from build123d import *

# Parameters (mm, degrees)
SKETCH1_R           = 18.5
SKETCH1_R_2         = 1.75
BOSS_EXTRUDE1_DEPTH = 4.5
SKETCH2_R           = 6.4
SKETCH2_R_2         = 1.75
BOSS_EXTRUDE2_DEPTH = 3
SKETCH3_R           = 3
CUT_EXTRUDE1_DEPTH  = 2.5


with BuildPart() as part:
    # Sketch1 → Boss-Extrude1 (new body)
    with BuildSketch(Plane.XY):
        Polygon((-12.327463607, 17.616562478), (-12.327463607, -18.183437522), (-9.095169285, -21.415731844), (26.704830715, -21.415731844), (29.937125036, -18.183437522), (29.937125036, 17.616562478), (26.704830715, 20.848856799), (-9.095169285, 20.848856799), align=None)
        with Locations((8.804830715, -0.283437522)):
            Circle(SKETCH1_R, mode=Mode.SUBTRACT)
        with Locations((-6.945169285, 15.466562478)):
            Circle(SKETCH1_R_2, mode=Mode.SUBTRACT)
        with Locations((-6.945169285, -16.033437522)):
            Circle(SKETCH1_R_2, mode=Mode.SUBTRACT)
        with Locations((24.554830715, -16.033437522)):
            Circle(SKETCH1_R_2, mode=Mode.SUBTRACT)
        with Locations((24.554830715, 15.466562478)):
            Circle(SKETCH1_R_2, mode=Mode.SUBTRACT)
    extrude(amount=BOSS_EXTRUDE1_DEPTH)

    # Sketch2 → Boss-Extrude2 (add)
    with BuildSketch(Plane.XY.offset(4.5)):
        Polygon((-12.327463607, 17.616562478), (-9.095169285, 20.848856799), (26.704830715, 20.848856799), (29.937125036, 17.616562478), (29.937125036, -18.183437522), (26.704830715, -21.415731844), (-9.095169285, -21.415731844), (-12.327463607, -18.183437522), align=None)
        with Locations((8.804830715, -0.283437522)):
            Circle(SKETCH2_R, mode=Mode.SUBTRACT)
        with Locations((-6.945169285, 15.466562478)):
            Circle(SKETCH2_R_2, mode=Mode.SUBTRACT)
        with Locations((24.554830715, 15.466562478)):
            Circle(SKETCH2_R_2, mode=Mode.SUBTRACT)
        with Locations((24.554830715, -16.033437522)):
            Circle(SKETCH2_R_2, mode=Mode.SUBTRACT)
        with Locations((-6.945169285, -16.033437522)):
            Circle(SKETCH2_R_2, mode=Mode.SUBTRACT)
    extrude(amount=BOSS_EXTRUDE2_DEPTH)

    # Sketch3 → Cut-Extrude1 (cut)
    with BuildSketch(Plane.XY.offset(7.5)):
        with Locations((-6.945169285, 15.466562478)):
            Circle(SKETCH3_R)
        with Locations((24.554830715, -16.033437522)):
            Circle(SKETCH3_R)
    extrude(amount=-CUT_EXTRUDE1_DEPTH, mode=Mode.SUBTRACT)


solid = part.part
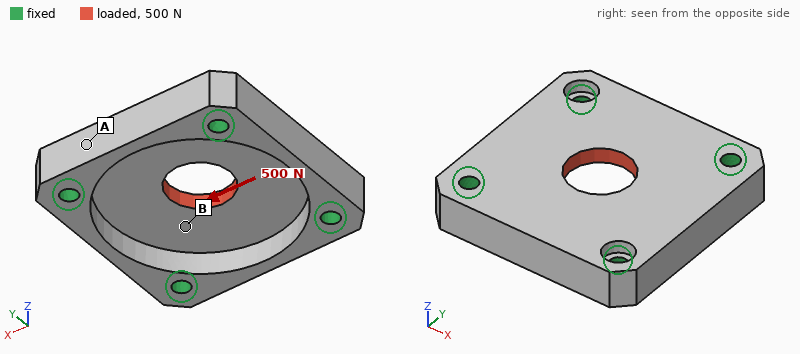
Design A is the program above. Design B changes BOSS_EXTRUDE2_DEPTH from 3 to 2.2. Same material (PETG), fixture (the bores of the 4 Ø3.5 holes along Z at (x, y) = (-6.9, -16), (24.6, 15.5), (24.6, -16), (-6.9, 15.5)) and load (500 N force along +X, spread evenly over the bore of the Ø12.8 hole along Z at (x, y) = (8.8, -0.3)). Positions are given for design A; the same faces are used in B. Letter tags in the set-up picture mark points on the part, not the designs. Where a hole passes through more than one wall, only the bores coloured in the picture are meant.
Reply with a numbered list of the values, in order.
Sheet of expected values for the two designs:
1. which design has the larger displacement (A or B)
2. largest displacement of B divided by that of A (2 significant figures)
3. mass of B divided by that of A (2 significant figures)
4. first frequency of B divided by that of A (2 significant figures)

1. B
2. 1.3
3. 0.84
4. 0.85
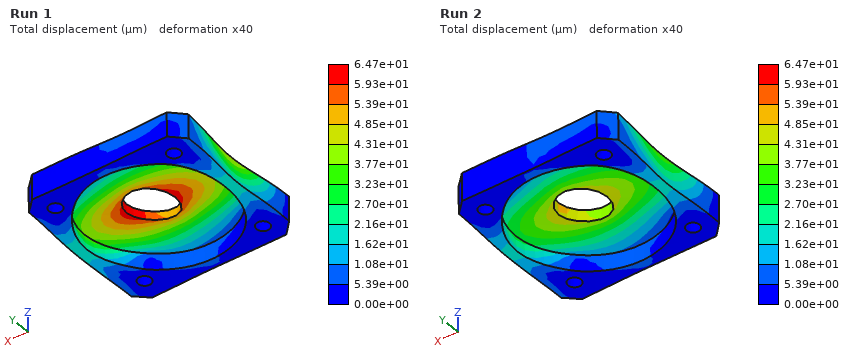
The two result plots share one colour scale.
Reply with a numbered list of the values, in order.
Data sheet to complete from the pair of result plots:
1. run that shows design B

1. Run 1
